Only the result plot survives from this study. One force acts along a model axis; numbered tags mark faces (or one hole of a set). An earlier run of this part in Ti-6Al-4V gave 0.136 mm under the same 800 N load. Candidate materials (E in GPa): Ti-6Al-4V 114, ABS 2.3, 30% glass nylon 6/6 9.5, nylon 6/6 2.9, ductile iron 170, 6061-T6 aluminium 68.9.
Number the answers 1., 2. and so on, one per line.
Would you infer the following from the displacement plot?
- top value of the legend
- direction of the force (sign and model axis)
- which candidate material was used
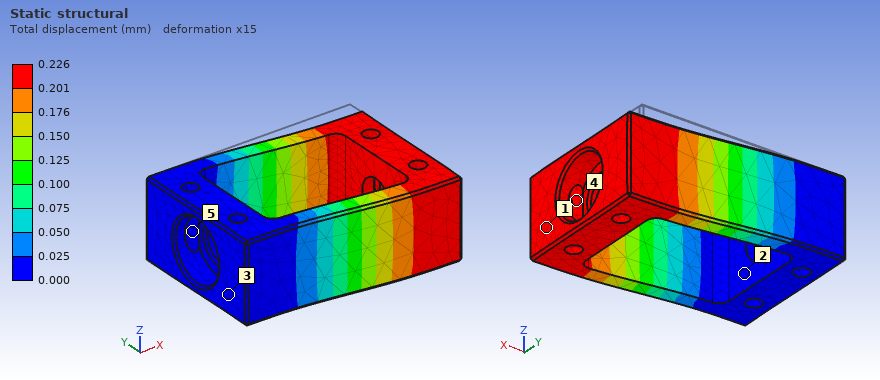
1. 0.226 mm
2. -Y
3. 6061-T6 aluminium
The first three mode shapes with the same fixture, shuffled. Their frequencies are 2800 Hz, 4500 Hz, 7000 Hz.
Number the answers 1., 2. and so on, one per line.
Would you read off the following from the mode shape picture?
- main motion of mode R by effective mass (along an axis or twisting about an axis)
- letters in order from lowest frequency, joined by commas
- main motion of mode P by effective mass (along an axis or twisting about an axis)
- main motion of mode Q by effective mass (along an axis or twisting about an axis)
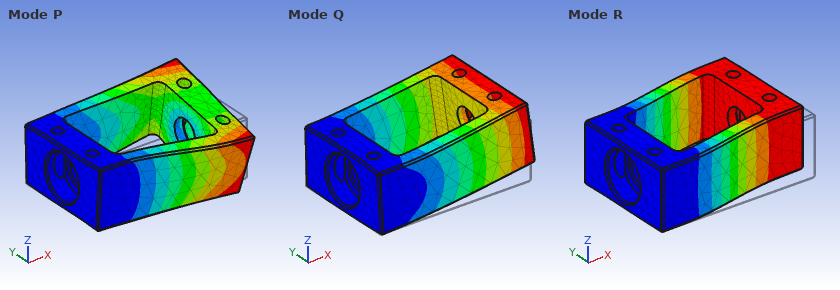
1. along Y
2. R, Q, P
3. twisting about X
4. along Z
